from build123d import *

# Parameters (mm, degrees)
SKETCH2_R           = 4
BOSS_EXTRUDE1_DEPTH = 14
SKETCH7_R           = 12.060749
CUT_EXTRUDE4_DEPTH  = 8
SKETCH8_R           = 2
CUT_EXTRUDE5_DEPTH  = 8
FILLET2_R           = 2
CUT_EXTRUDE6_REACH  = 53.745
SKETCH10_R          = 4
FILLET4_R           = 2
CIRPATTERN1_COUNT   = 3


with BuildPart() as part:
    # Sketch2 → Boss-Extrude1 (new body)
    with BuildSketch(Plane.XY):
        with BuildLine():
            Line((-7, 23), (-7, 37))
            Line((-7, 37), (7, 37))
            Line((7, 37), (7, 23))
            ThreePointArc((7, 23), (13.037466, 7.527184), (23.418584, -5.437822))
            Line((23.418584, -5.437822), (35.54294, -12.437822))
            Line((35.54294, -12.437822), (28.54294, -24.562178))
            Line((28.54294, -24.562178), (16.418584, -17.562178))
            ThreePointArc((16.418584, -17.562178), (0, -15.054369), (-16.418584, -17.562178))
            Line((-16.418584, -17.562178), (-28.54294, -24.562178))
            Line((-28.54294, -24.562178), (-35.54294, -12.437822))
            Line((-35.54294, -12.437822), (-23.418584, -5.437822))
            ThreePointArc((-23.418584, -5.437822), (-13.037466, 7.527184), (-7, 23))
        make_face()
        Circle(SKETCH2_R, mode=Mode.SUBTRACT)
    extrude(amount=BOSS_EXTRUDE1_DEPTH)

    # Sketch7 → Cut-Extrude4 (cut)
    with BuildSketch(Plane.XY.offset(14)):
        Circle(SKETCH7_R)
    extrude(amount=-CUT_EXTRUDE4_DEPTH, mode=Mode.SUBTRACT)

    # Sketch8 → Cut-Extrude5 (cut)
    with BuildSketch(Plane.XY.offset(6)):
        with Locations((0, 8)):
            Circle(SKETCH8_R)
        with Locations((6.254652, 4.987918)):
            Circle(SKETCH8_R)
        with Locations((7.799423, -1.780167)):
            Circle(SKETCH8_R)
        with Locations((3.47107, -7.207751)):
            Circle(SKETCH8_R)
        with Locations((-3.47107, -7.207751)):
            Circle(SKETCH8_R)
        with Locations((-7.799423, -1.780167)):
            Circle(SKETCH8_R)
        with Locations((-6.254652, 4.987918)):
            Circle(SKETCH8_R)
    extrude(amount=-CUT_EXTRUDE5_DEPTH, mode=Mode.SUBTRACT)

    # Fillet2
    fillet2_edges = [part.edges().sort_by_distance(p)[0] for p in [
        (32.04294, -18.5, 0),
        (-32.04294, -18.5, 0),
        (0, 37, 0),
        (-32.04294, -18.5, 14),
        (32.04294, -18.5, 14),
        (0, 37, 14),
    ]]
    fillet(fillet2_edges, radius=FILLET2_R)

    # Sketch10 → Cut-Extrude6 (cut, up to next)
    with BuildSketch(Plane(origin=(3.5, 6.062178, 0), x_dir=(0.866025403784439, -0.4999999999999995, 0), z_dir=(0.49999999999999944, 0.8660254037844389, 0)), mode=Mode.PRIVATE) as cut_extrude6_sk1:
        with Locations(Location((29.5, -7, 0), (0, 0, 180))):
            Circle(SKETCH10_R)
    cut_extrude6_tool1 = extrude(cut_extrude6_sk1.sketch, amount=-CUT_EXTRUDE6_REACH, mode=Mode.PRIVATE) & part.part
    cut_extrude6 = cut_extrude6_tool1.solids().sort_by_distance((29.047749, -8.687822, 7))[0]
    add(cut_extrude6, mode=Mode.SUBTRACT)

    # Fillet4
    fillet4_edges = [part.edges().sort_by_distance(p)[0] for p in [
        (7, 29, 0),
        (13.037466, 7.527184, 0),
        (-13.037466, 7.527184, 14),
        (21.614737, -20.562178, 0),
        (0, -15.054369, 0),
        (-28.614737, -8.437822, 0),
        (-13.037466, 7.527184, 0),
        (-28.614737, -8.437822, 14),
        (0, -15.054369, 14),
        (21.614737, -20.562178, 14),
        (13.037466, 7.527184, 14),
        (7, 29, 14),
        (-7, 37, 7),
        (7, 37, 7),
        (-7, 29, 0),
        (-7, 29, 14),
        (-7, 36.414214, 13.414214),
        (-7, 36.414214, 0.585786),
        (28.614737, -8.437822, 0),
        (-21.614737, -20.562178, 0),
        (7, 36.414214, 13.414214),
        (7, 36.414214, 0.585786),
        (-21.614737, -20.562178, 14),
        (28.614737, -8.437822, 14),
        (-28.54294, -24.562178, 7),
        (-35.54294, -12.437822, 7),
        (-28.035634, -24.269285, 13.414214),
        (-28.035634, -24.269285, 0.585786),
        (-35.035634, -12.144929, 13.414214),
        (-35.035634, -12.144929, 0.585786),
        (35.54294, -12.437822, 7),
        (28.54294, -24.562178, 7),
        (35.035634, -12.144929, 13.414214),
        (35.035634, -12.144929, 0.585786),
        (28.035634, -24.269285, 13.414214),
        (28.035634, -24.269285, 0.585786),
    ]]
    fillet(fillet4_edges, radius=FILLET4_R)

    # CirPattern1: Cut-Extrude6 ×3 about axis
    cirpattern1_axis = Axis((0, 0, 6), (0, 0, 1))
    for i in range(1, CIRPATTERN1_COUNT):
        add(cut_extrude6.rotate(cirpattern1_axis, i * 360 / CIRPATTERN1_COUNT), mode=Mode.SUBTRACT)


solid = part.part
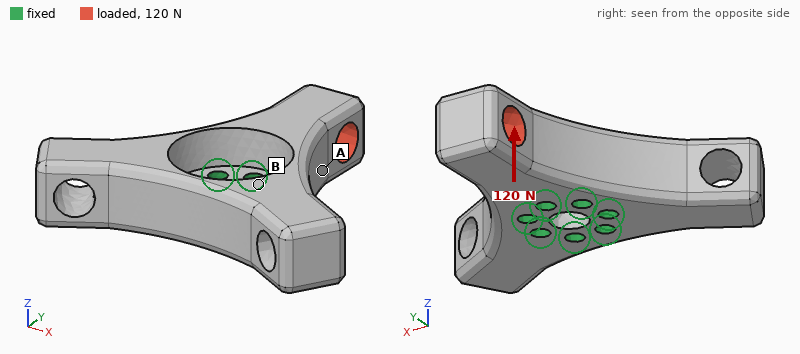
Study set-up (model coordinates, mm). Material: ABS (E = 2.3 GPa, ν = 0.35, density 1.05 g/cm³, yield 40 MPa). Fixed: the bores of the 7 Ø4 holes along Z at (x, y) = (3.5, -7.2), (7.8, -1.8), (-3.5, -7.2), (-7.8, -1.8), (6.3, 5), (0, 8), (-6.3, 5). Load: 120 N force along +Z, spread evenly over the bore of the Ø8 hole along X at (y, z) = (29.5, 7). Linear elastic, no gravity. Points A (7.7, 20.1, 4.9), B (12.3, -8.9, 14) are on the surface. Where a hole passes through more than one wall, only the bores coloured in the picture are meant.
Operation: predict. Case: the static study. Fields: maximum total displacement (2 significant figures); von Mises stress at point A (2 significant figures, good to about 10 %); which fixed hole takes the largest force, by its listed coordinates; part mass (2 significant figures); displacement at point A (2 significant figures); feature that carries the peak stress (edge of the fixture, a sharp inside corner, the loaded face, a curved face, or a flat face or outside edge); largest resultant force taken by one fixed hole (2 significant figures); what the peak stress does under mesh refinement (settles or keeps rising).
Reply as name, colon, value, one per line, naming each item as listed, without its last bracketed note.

maximum total displacement: 0.25 mm
von Mises stress at point A: 2.2 MPa
which fixed hole takes the largest force, by its listed coordinates: (0, 8)
part mass: 19 g
displacement at point A: 0.076 mm
feature that carries the peak stress: edge of the fixture
largest resultant force taken by one fixed hole: 150 N
what the peak stress does under mesh refinement: keeps rising
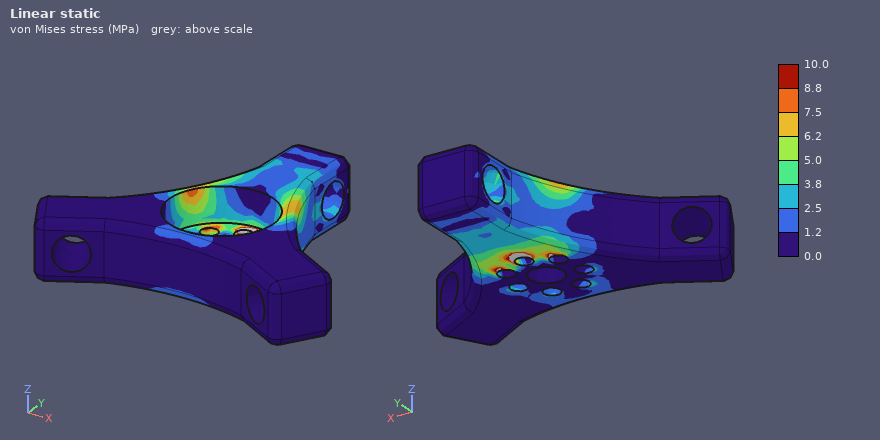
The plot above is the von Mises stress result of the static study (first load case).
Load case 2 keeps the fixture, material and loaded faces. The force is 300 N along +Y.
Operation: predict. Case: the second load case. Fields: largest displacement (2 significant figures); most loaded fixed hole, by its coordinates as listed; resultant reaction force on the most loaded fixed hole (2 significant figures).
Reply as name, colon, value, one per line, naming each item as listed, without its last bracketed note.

largest displacement: 87 µm
most loaded fixed hole, by its coordinates as listed: (0, 8)
resultant reaction force on the most loaded fixed hole: 99 N
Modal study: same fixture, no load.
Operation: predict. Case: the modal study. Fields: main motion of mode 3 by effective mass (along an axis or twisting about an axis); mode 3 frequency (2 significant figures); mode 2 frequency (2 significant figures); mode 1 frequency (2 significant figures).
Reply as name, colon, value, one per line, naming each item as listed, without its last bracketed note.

main motion of mode 3 by effective mass: along Z
mode 3 frequency: 3000 Hz
mode 2 frequency: 2300 Hz
mode 1 frequency: 2300 Hz
